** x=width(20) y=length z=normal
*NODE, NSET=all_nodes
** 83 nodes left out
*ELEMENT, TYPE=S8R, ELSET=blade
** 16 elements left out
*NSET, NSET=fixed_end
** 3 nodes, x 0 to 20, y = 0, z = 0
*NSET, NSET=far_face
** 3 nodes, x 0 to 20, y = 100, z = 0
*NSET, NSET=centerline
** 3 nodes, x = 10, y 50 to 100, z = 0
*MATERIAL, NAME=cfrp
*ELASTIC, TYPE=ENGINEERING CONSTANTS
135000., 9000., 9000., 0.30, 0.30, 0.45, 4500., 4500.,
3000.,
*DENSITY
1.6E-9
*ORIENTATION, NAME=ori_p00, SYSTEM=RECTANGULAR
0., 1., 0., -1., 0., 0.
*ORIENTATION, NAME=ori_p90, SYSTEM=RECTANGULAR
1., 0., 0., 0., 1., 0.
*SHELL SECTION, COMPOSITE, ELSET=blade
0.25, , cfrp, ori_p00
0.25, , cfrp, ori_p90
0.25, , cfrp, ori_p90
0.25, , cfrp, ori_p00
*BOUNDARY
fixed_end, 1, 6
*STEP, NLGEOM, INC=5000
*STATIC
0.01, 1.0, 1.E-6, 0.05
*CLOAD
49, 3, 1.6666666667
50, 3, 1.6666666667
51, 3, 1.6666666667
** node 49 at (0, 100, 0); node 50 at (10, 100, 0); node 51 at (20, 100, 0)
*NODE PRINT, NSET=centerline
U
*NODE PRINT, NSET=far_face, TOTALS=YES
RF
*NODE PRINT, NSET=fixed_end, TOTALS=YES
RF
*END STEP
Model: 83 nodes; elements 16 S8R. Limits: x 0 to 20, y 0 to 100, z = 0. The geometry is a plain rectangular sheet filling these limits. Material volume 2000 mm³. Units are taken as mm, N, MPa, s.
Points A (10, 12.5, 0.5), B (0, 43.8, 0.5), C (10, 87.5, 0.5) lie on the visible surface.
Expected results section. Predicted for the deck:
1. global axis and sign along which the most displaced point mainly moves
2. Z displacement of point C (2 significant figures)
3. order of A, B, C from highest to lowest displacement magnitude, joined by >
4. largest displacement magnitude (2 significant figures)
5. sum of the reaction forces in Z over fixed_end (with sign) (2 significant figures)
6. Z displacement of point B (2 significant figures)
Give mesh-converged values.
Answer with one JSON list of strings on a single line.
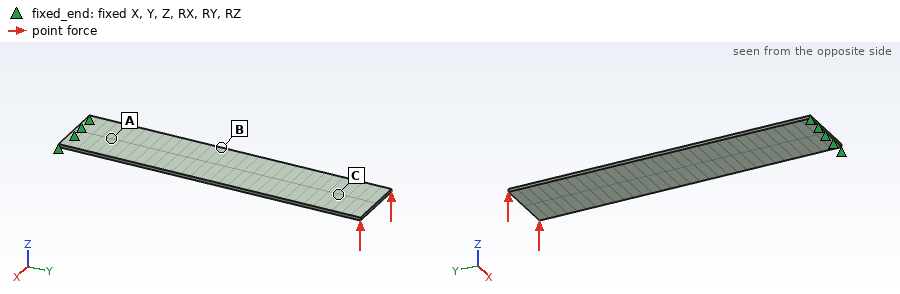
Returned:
["+Z", "6.7 mm", "C > B > A", "8.3 mm", "-5.0 N", "2.0 mm"]
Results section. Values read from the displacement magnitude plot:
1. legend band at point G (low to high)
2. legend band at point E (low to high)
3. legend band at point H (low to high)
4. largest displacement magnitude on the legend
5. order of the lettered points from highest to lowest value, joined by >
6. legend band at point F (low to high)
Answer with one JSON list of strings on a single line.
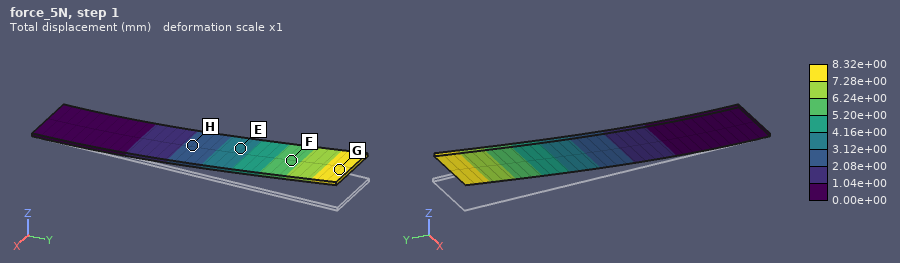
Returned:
["7.28e+00 to 8.32e+00 mm", "3.12e+00 to 4.16e+00 mm", "2.08e+00 to 3.12e+00 mm", "8.32e+00 mm", "G > F > E > H", "5.20e+00 to 6.24e+00 mm"]
